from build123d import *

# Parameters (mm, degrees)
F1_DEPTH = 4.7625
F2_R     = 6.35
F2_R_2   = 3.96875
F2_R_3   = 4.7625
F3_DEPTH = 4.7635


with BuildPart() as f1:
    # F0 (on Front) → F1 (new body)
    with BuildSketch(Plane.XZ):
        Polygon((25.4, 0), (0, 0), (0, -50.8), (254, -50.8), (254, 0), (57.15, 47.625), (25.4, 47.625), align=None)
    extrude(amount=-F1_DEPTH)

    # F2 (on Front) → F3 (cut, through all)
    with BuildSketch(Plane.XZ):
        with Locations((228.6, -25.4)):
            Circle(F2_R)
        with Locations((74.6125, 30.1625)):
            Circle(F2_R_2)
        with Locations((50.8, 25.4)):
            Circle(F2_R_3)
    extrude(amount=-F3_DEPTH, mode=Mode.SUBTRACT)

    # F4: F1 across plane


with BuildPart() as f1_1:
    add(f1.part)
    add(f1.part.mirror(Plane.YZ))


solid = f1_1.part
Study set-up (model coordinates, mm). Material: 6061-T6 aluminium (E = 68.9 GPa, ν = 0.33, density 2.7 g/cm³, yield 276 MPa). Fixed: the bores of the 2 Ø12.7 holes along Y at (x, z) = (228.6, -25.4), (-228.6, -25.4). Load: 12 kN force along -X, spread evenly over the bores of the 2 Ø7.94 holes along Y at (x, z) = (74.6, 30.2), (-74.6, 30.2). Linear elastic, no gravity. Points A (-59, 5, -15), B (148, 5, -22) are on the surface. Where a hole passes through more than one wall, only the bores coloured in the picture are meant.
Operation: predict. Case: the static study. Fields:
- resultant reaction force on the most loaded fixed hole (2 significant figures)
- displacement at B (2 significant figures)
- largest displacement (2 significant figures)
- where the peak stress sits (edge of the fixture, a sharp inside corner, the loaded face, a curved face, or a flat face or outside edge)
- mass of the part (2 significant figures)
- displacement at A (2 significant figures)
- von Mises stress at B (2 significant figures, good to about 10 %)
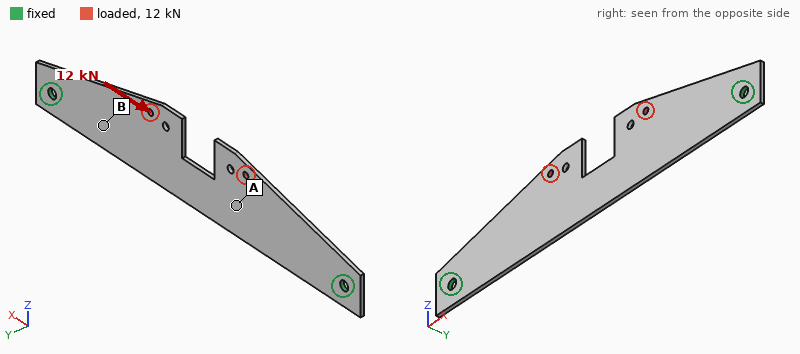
6.2 kN
27 µm
72 µm
the loaded face
480 g
39 µm
15 MPa
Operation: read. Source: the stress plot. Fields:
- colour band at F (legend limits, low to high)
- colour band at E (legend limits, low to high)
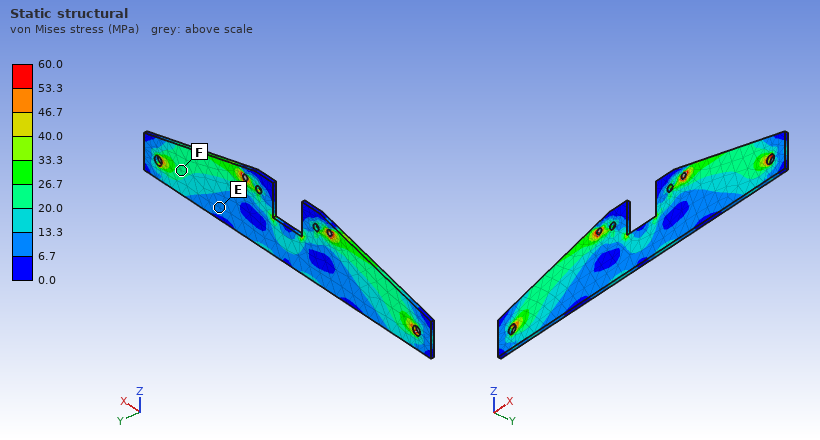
20.0 to 26.7 MPa
6.7 to 13.3 MPa
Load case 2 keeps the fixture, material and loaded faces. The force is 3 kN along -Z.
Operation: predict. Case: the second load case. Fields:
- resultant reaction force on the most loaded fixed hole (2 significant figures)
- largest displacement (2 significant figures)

1.6 kN
0.43 mm
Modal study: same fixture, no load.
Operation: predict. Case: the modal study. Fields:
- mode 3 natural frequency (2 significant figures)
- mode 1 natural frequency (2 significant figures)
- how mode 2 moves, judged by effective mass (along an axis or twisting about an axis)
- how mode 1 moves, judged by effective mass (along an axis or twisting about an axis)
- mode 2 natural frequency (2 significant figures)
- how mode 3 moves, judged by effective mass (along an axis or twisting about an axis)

330 Hz
110 Hz
twisting about Z
along Y
290 Hz
twisting about X
